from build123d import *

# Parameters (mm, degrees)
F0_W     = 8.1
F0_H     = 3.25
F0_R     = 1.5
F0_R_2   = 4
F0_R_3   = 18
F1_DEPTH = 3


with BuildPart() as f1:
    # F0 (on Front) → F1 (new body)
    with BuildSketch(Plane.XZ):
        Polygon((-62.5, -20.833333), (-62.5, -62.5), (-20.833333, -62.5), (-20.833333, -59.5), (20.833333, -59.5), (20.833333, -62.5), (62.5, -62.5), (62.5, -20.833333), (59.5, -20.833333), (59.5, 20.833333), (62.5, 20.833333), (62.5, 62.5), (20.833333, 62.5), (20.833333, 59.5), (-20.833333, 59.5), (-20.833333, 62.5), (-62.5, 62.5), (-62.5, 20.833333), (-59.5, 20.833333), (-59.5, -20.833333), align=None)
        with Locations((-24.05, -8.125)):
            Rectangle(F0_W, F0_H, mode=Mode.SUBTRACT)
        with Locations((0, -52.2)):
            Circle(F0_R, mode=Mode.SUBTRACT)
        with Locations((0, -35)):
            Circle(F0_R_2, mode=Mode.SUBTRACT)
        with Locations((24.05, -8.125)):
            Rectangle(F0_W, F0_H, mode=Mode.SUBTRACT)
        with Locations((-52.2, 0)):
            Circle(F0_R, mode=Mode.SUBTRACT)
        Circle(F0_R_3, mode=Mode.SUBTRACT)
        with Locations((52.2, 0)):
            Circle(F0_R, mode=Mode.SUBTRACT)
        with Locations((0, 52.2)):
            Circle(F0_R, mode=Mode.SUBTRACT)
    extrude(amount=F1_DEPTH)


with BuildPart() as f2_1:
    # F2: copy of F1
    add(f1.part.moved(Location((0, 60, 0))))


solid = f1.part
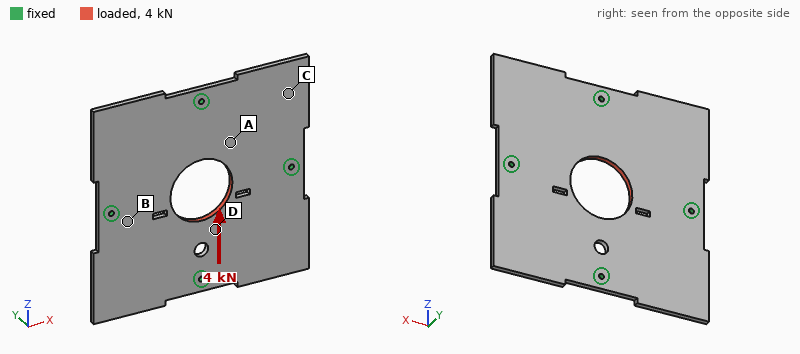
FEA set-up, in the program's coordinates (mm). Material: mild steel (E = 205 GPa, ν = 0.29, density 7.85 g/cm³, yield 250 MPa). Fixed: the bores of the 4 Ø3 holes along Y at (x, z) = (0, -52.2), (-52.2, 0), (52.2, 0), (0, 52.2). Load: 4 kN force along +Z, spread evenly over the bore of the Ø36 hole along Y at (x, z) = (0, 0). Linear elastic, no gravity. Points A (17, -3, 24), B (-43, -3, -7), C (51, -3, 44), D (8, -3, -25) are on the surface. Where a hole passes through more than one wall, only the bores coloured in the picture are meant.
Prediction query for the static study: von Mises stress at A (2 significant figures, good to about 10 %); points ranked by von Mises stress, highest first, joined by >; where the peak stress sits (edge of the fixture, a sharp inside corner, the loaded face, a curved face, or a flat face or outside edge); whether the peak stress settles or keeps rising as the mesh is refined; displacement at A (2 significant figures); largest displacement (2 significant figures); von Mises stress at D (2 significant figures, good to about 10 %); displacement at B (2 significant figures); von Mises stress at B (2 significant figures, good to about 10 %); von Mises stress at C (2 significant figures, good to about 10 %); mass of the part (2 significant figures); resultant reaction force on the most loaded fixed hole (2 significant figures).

11 MPa
D > A > B > C
edge of the fixture
keeps rising
2.7 µm
3.8 µm
16 MPa
1.3 µm
6.7 MPa
2.8 MPa
330 g
1.2 kN
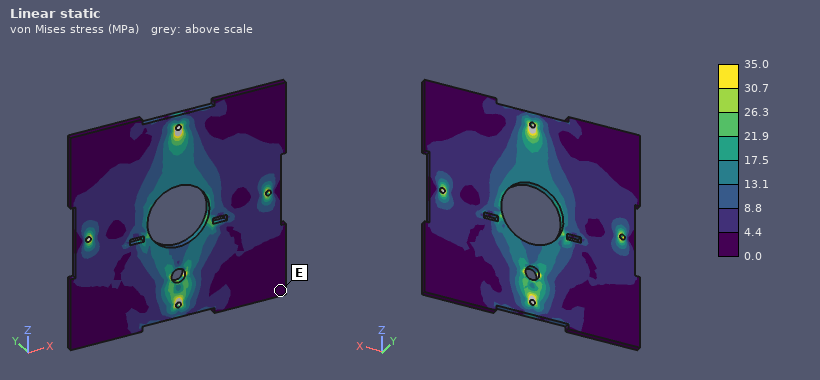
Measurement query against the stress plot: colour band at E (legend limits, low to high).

0.0 to 4.4 MPa
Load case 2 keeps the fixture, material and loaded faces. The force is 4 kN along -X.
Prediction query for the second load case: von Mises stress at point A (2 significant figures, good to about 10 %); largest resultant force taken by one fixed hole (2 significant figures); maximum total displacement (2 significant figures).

8.1 MPa
1.1 kN
3.6 µm
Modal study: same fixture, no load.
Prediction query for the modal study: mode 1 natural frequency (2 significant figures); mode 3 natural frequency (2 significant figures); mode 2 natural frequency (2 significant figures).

1100 Hz
1200 Hz
1200 Hz
